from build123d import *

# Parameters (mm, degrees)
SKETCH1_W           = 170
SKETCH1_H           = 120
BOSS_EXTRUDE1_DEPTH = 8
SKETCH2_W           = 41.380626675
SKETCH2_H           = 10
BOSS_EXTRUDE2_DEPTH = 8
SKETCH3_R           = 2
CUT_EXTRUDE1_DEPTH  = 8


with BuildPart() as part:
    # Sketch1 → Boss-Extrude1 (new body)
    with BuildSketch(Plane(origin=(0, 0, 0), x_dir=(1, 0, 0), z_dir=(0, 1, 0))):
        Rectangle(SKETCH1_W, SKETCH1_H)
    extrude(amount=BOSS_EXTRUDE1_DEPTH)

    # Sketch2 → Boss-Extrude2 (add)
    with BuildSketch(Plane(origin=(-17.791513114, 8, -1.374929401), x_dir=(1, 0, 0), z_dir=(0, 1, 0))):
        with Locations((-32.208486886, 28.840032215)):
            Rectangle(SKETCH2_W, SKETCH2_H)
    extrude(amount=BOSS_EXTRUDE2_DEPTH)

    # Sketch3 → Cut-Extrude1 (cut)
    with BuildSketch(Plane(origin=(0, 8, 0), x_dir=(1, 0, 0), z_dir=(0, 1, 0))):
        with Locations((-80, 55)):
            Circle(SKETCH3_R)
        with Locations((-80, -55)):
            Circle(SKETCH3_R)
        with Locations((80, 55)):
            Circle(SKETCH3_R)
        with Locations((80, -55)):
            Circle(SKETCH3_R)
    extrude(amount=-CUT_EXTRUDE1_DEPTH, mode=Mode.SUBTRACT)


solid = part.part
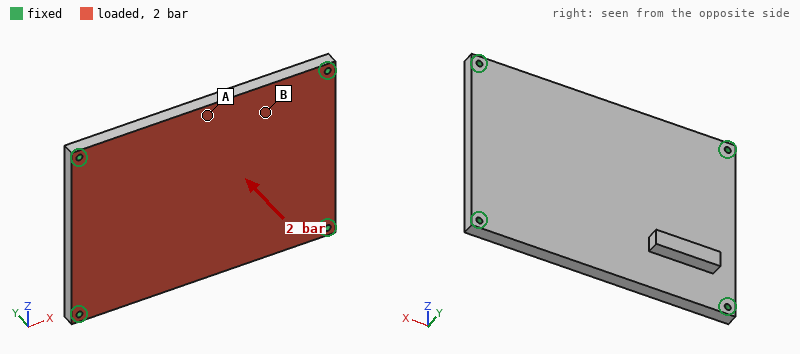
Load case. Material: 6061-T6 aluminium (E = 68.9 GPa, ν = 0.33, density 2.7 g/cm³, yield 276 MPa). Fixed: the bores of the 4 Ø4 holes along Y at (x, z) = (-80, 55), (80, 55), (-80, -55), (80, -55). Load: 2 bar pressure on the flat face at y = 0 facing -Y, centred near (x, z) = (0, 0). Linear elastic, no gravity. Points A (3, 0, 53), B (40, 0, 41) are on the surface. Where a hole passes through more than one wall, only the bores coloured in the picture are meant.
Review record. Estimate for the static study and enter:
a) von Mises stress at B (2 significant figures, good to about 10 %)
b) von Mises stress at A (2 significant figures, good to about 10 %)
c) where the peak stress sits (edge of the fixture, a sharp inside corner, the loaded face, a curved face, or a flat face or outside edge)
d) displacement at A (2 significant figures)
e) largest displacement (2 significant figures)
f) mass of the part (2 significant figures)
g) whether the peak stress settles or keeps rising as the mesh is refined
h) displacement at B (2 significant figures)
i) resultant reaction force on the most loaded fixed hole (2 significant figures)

17 MPa
32 MPa
edge of the fixture
0.23 mm
0.25 mm
450 g
keeps rising
0.16 mm
1.0 kN
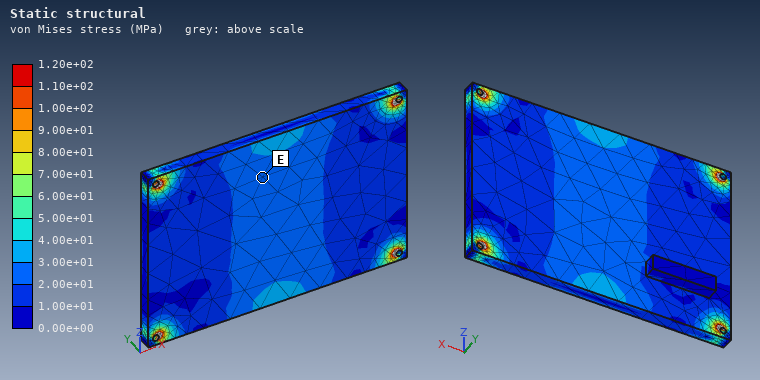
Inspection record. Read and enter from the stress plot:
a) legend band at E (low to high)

2.00e+01 to 3.00e+01 MPa
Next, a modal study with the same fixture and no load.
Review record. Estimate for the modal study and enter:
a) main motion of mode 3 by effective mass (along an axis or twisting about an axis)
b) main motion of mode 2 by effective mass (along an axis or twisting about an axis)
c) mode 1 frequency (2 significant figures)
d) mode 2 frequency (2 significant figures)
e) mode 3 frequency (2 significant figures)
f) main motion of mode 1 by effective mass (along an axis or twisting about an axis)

twisting about Z
twisting about X
1100 Hz
2000 Hz
2700 Hz
along Y
